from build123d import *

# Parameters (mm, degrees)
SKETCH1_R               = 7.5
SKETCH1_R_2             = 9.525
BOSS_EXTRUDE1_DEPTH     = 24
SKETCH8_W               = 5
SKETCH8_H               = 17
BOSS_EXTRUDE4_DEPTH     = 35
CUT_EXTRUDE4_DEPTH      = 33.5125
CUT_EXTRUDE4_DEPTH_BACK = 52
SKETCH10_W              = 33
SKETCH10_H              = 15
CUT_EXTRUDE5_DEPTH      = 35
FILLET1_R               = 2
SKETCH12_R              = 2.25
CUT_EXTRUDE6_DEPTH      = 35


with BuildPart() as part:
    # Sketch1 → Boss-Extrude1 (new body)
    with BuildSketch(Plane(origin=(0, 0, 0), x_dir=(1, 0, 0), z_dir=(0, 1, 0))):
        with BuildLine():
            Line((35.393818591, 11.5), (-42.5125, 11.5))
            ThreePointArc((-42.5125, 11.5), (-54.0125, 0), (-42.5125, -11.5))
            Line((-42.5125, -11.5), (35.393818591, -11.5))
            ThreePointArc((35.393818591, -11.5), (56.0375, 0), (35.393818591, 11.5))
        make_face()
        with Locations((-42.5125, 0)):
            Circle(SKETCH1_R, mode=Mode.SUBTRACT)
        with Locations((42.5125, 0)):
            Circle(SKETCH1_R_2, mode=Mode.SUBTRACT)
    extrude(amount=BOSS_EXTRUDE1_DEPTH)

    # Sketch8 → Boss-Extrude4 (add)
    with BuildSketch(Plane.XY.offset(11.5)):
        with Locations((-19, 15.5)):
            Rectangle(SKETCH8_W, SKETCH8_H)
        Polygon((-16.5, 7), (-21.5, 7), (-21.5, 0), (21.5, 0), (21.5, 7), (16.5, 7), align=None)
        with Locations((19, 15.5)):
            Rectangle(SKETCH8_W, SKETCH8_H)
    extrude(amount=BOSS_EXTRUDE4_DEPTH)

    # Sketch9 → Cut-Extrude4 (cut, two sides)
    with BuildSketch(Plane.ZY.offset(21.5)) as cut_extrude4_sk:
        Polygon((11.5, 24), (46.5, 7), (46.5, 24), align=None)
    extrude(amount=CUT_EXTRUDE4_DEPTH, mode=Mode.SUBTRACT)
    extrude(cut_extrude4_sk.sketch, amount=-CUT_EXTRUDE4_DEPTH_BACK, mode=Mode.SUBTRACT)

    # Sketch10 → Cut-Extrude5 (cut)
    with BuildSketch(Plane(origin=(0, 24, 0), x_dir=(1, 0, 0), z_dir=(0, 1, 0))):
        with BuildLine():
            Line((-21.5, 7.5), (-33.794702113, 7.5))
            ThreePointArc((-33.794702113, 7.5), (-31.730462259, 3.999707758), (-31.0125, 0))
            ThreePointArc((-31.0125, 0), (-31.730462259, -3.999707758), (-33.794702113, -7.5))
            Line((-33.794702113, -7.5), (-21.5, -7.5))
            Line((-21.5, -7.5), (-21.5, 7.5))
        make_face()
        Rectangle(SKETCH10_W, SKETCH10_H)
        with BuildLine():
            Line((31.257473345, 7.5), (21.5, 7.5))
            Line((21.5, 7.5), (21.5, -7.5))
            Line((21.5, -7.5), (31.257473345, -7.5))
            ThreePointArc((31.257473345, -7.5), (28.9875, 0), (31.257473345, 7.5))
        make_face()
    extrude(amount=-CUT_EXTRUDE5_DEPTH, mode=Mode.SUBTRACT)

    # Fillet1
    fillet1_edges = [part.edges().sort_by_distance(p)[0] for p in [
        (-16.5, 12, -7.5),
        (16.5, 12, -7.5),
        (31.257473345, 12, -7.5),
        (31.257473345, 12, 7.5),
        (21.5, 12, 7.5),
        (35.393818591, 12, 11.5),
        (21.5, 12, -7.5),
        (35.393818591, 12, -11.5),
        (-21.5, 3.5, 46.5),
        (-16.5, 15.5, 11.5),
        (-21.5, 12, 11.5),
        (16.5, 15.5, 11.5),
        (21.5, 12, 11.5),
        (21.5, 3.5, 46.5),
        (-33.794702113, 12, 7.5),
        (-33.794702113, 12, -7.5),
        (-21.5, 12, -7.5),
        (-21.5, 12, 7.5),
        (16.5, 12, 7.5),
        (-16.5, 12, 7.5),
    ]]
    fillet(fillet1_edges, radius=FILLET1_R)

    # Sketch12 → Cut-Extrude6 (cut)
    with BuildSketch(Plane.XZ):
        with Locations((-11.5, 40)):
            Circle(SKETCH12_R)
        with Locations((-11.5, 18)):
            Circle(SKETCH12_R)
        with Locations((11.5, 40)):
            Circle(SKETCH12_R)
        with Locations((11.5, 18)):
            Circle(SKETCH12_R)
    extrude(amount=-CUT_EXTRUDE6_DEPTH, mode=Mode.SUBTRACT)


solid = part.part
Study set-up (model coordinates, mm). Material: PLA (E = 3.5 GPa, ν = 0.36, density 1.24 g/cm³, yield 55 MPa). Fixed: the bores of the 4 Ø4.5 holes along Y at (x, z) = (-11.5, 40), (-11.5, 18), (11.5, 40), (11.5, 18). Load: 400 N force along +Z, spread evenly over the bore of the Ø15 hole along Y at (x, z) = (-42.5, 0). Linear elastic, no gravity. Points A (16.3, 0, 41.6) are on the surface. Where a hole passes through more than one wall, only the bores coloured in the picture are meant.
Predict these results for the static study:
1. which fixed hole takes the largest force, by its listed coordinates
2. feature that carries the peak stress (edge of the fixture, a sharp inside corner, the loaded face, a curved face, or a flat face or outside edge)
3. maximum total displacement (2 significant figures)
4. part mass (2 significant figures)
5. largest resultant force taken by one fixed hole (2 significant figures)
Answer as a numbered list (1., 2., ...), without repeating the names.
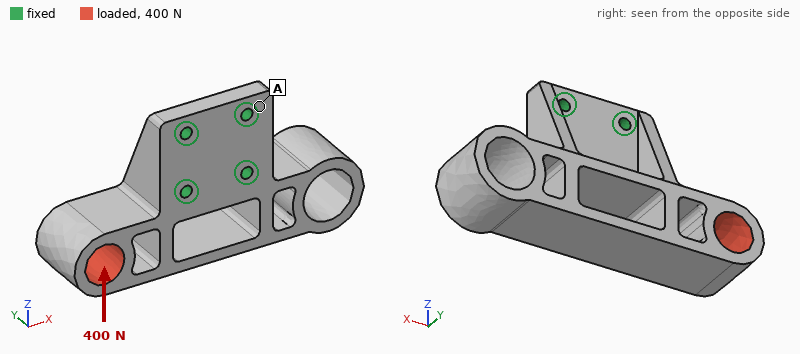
1. (-11.5, 18)
2. a curved face
3. 0.86 mm
4. 54 g
5. 390 N
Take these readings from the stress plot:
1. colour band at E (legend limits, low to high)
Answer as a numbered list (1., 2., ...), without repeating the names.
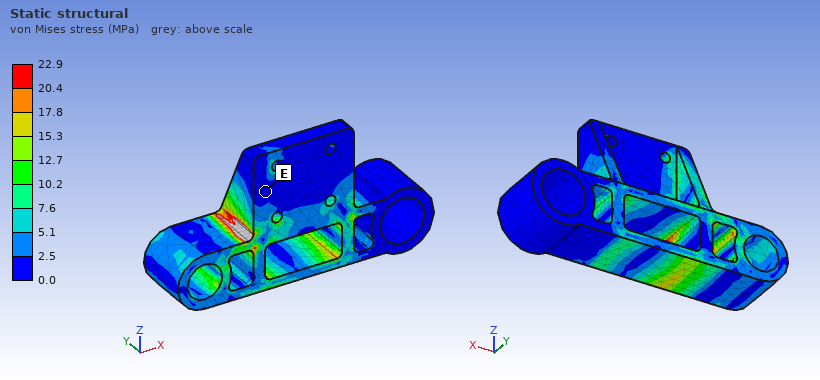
1. 0.0 to 2.5 MPa
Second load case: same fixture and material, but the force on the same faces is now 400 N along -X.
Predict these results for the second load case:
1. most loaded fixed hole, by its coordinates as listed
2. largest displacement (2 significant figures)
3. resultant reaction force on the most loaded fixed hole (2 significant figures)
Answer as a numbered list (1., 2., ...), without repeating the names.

1. (-11.5, 18)
2. 0.30 mm
3. 310 N
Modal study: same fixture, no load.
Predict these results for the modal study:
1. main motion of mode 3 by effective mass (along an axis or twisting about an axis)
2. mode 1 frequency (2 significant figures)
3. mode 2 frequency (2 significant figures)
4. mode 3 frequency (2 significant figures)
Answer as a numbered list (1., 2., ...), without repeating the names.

1. along Y
2. 900 Hz
3. 950 Hz
4. 1300 Hz
